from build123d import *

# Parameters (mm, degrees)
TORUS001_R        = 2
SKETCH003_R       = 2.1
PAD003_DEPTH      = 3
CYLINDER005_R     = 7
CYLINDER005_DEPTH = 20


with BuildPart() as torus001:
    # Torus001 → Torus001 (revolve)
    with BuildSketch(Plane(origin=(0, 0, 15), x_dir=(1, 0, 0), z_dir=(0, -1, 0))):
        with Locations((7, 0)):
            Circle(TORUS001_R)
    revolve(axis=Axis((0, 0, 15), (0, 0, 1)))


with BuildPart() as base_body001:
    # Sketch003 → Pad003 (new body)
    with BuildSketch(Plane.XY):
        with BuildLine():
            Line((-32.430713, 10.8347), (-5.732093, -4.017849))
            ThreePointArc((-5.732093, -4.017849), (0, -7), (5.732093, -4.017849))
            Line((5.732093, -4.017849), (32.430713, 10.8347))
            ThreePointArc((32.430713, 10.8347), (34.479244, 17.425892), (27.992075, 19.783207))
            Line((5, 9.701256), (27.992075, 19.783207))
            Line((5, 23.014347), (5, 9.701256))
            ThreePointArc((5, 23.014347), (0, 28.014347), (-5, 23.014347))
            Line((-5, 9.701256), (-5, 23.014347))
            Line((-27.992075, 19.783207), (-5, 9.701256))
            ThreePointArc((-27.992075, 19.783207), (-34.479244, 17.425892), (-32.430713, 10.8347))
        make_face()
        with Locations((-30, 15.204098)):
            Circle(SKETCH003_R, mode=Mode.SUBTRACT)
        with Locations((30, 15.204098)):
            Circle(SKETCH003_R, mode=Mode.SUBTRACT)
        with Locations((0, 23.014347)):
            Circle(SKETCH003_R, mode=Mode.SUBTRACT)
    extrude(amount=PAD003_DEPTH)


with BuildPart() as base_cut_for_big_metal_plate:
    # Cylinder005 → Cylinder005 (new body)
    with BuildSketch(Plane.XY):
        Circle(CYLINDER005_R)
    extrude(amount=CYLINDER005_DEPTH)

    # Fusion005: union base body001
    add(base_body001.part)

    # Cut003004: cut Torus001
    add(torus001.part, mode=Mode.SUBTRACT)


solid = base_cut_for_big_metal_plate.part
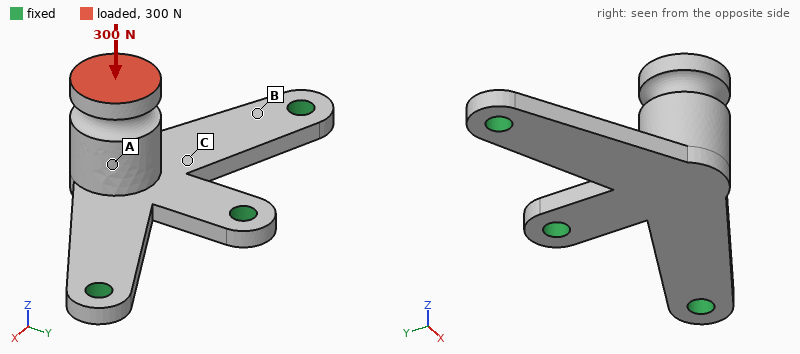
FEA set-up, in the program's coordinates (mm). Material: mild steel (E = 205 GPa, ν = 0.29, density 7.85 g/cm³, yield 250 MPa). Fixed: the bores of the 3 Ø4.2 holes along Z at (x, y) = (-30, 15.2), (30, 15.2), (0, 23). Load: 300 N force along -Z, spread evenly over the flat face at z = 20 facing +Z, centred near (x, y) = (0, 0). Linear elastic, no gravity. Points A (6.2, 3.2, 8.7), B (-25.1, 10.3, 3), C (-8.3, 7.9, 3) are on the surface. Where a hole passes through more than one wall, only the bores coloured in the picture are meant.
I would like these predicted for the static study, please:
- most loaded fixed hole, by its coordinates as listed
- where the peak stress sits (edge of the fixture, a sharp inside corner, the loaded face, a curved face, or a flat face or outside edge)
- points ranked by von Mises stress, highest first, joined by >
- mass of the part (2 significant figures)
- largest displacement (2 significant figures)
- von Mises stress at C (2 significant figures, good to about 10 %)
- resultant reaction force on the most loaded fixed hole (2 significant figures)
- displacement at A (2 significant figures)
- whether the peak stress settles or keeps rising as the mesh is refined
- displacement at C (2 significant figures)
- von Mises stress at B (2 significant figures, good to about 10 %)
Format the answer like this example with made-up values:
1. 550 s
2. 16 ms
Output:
1. (0, 23)
2. edge of the fixture
3. B > C > A
4. 42 g
5. 0.12 mm
6. 46 MPa
7. 130 N
8. 0.060 mm
9. keeps rising
10. 0.033 mm
11. 84 MPa
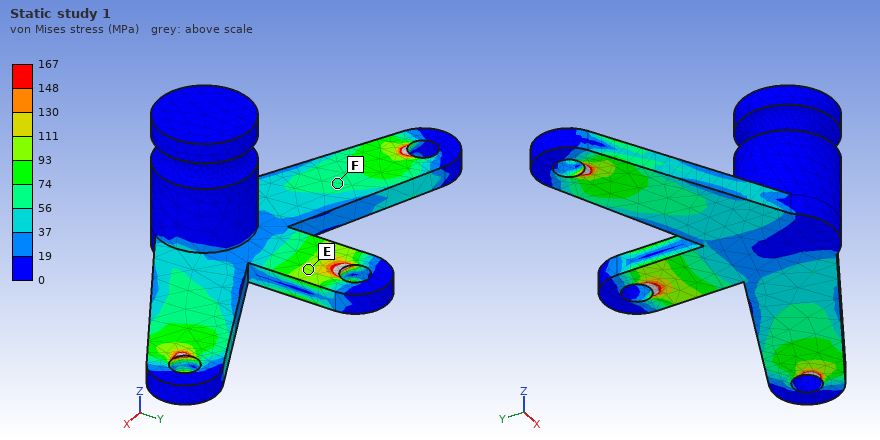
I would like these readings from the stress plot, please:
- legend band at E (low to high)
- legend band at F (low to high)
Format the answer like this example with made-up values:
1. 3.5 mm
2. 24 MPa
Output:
1. 93 to 111 MPa
2. 56 to 74 MPa
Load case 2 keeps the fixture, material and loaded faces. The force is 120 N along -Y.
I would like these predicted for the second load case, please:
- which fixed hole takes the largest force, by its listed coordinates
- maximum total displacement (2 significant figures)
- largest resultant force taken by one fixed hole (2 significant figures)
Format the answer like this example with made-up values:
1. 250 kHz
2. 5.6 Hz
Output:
1. (0, 23)
2. 68 µm
3. 130 N
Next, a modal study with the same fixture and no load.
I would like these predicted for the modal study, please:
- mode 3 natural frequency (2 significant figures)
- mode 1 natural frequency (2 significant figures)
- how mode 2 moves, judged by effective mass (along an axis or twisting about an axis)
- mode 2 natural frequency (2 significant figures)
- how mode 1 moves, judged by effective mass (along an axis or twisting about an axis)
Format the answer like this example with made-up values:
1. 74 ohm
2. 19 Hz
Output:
1. 6400 Hz
2. 1800 Hz
3. along X
4. 4700 Hz
5. along Z
